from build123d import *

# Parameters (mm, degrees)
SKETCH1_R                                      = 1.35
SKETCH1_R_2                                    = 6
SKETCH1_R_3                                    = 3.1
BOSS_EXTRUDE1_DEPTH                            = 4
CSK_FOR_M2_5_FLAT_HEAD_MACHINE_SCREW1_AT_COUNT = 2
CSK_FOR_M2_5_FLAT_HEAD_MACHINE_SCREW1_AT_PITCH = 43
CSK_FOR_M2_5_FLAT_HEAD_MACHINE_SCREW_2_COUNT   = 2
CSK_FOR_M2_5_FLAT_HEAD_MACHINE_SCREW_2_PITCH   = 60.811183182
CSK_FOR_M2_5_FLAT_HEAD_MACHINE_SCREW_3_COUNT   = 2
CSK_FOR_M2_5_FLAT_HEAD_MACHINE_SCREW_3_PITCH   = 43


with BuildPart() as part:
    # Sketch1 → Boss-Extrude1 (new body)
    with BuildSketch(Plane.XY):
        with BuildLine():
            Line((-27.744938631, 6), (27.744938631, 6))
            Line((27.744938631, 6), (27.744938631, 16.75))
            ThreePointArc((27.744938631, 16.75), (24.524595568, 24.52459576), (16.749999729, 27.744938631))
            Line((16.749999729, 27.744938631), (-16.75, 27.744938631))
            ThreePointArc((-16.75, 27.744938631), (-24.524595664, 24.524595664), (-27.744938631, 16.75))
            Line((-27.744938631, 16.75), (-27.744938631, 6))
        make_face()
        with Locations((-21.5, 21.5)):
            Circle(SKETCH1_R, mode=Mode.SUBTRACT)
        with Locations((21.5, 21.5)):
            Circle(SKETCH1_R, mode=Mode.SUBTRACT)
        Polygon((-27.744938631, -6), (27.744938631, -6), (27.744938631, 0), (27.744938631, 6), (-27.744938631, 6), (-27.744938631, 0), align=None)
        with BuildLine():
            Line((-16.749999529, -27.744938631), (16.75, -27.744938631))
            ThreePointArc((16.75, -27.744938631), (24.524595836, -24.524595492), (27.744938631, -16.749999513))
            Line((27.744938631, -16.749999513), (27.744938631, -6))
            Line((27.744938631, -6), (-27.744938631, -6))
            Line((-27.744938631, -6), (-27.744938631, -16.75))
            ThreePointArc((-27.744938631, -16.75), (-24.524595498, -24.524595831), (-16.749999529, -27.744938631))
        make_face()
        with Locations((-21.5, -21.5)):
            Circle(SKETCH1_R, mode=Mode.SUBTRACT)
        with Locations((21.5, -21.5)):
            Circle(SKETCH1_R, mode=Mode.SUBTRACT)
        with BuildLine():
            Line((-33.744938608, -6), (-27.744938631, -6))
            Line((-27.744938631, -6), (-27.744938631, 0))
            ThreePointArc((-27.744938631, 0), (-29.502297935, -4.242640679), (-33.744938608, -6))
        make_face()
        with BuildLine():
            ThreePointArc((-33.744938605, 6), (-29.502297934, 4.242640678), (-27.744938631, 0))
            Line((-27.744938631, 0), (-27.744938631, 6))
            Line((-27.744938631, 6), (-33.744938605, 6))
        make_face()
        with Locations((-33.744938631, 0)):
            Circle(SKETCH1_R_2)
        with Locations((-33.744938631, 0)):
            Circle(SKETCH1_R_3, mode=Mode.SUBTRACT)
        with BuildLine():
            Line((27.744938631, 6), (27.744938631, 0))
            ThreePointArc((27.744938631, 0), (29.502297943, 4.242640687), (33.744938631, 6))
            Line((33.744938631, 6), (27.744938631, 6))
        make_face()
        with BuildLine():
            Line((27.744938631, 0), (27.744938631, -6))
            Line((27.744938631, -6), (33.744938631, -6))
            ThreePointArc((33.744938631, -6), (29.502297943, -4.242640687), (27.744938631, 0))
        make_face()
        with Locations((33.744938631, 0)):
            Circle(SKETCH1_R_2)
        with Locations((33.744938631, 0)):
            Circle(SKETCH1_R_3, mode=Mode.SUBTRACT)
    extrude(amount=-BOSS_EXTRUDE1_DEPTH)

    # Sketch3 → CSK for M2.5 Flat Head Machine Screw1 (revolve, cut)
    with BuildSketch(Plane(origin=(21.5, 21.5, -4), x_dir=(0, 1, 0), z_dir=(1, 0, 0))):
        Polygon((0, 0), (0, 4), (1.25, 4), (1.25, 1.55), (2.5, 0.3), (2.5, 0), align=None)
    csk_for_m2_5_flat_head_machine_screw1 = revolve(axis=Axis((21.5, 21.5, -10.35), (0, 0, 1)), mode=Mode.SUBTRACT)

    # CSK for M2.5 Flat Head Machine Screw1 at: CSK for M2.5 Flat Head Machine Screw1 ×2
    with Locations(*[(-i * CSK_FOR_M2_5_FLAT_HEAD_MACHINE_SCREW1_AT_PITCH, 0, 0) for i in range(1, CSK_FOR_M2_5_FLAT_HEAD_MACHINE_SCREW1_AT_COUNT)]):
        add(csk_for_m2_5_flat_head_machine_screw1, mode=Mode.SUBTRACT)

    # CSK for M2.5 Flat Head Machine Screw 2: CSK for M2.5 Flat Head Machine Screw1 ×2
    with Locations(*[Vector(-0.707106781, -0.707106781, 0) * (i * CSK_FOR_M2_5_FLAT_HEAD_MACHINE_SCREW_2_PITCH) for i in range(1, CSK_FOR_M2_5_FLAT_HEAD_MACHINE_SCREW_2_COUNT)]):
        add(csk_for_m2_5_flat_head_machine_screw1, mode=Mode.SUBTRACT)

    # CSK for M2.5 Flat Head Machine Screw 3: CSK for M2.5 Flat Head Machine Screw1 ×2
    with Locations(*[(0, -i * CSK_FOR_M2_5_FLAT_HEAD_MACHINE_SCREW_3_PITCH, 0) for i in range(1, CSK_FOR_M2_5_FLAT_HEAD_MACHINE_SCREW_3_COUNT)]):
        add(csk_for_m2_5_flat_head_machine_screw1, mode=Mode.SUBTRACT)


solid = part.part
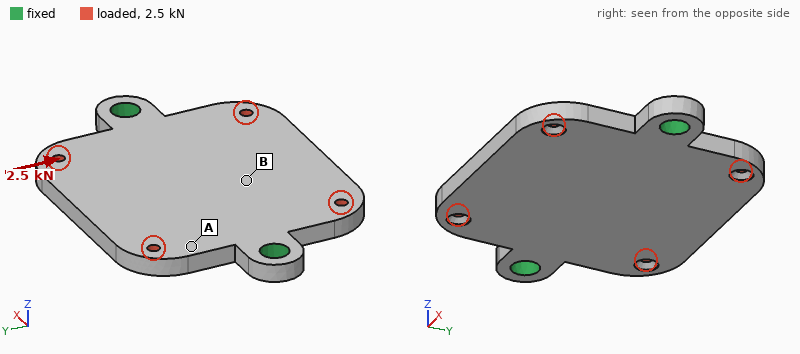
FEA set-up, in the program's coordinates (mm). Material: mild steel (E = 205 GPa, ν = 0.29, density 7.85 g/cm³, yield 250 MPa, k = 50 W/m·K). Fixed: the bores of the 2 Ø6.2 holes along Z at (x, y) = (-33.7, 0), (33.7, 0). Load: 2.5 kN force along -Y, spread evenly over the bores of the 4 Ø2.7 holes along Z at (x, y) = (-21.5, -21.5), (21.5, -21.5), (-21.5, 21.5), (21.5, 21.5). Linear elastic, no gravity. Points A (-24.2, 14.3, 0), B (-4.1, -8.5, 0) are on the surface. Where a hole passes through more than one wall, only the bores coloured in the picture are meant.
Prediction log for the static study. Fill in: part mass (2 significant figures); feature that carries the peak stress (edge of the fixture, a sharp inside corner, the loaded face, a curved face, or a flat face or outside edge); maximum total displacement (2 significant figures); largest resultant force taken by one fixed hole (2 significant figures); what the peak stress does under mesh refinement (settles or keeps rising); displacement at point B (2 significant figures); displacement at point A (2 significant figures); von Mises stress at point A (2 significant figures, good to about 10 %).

99 g
edge of the fixture
17 µm
1.3 kN
keeps rising
6.4 µm
7.5 µm
27 MPa
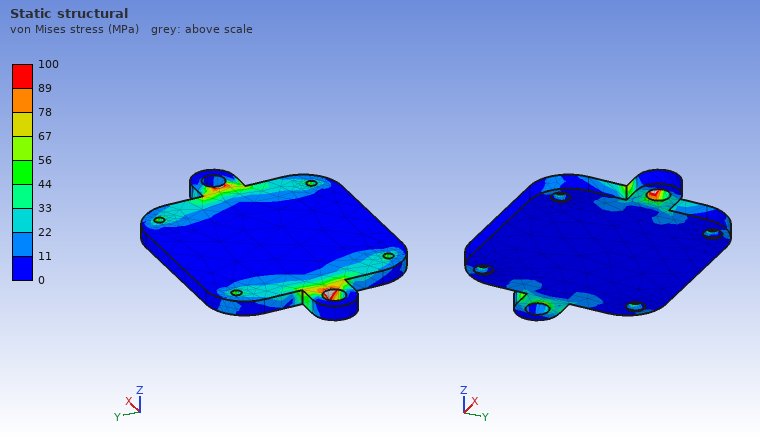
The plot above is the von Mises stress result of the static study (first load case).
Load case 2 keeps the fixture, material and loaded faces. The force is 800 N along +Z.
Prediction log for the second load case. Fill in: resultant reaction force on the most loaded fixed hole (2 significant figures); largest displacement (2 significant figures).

400 N
41 µm
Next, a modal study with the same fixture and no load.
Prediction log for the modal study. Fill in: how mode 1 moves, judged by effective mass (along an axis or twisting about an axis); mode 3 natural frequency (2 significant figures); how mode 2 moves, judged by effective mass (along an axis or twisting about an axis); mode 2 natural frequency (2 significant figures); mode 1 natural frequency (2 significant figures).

twisting about X
6300 Hz
along Z
2900 Hz
2100 Hz
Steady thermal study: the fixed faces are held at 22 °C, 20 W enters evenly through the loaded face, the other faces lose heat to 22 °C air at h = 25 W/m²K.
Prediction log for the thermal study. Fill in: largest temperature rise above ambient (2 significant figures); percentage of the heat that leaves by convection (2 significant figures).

51 K
28 %
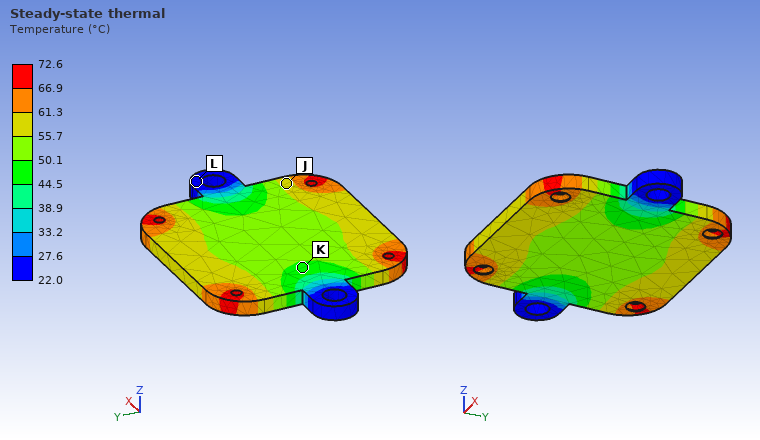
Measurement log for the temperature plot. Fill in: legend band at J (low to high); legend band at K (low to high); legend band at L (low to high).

55.7 to 61.3 °C
44.5 to 50.1 °C
22.0 to 27.6 °C
